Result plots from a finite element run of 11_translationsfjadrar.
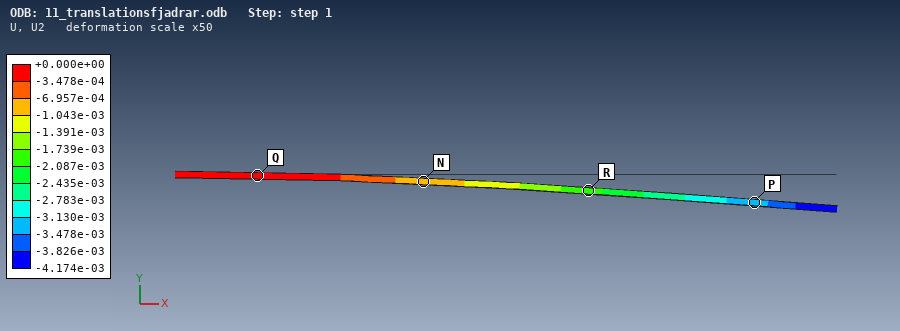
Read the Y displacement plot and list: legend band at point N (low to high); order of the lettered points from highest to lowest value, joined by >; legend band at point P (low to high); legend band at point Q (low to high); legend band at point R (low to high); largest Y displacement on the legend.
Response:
-1.043e-03 to -6.957e-04
Q > N > R > P
-3.478e-03 to -3.130e-03
-3.478e-04 to +0.000e+00
-2.087e-03 to -1.739e-03
+0.000e+00
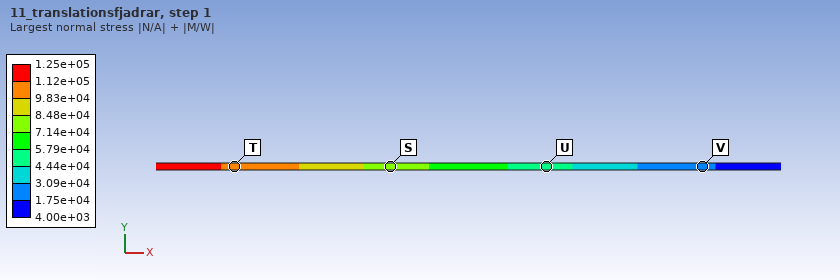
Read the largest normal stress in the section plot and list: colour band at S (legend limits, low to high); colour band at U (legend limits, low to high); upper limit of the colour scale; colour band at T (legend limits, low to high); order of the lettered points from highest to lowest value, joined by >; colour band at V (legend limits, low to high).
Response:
7.14e+04 to 8.48e+04
4.44e+04 to 5.79e+04
1.25e+05
9.83e+04 to 1.12e+05
T > S > U > V
1.75e+04 to 3.09e+04
